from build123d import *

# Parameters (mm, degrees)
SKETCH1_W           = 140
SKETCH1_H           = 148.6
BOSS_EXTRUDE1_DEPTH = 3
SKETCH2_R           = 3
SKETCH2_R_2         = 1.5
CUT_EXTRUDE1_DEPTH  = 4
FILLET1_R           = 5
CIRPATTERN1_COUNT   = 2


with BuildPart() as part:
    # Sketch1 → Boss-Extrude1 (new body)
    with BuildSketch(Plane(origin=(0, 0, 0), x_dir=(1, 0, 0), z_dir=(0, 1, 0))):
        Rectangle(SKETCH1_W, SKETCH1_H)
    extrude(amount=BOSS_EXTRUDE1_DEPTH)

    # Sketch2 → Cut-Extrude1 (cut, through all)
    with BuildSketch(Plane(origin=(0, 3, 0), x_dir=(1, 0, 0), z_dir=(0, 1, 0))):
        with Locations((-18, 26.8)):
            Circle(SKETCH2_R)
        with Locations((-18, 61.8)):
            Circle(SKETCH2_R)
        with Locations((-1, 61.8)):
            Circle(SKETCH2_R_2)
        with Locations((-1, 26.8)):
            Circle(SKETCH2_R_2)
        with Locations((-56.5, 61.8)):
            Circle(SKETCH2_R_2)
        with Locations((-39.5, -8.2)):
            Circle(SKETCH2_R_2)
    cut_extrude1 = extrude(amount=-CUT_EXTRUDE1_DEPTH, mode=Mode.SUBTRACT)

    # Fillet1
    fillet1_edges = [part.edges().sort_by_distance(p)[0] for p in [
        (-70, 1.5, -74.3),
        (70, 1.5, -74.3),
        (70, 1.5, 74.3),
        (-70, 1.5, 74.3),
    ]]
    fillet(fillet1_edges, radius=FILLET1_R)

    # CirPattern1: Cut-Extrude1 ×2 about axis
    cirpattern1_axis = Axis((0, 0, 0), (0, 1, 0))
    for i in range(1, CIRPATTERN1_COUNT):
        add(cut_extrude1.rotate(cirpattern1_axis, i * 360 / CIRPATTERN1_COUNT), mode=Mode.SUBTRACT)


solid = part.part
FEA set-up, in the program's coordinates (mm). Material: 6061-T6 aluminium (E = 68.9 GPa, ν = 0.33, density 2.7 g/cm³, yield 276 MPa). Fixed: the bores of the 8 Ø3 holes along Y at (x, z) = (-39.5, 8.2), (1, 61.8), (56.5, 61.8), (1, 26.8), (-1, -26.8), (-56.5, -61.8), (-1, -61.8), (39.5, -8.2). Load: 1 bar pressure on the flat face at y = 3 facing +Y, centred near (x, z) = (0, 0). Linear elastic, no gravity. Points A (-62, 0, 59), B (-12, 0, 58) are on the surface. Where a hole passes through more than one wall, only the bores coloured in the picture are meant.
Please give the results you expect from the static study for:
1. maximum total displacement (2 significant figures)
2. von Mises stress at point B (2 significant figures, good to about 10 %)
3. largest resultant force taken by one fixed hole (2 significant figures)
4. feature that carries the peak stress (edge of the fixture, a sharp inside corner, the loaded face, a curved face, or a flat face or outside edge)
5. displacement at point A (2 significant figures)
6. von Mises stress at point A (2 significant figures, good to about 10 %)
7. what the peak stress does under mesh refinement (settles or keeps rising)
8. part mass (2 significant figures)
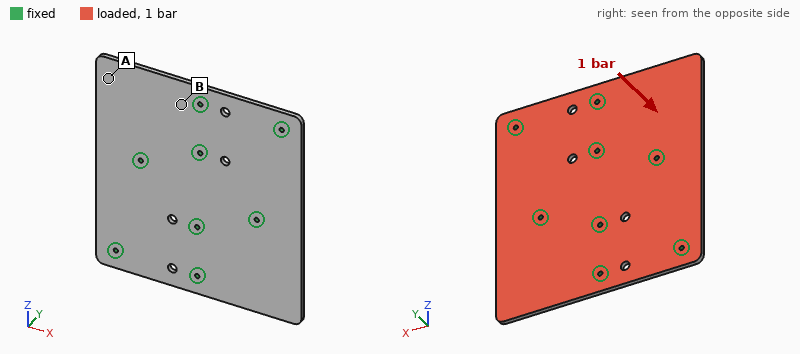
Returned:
0.73 mm
38 MPa
470 N
edge of the fixture
0.54 mm
14 MPa
keeps rising
170 g
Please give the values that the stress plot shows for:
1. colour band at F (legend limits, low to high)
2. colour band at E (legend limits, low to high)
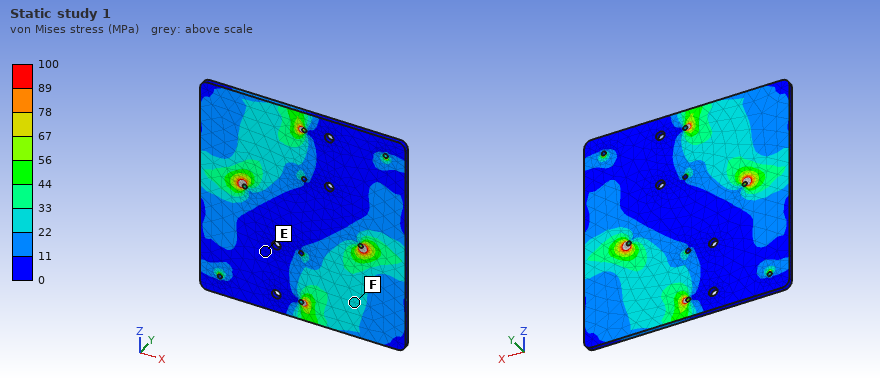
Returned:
22 to 33 MPa
0 to 11 MPa
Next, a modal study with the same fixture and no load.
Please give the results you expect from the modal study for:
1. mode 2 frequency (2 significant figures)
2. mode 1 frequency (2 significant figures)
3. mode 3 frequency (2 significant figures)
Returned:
920 Hz
910 Hz
2300 Hz
